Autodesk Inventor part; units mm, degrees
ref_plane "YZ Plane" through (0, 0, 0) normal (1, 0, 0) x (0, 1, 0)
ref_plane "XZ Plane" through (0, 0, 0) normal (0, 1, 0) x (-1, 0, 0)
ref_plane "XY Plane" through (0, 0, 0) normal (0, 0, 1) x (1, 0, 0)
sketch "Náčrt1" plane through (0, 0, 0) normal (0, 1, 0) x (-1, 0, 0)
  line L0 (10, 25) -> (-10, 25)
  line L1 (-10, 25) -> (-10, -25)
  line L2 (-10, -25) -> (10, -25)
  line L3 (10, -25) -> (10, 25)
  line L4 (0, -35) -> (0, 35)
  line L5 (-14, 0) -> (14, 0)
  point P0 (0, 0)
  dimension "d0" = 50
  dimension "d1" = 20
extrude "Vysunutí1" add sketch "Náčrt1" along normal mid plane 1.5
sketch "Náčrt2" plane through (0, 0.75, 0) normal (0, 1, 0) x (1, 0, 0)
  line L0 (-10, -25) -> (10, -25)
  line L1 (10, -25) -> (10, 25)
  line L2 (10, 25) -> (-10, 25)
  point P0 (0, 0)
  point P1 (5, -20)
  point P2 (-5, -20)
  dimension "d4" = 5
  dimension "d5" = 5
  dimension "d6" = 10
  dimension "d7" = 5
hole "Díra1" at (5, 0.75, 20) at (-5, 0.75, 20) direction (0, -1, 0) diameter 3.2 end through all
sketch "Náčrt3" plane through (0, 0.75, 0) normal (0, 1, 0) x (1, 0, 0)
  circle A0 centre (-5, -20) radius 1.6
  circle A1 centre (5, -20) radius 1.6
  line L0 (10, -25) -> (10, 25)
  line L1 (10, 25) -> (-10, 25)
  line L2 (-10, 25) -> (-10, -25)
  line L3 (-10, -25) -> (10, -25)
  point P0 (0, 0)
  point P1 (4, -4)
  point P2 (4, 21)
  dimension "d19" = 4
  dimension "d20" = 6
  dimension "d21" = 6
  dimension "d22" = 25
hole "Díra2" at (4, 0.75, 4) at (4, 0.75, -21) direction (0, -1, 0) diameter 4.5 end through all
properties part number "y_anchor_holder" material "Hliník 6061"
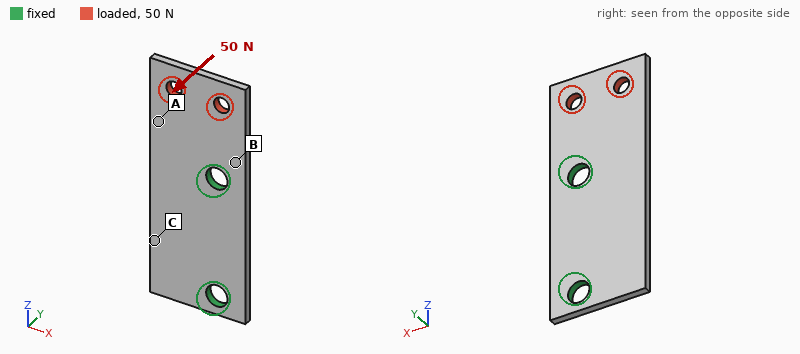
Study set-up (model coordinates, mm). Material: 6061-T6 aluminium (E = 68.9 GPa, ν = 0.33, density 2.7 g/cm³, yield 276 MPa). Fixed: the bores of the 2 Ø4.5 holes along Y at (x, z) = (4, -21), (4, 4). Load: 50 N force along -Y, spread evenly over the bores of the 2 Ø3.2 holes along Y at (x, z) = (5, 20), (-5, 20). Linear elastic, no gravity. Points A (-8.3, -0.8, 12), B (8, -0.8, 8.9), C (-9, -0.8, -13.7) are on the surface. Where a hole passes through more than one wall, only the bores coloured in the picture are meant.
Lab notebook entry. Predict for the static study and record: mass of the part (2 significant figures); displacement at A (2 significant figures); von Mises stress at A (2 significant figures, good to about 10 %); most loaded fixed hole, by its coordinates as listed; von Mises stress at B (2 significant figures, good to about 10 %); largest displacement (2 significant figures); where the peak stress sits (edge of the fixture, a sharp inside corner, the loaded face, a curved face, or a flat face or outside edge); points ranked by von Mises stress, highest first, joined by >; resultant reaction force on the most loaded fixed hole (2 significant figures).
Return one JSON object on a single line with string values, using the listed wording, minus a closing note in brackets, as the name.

{"mass of the part": "3.9 g", "displacement at A": "0.071 mm", "von Mises stress at A": "42 MPa", "most loaded fixed hole, by its coordinates as listed": "(4, 4)", "von Mises stress at B": "81 MPa", "largest displacement": "0.26 mm", "where the peak stress sits": "a flat face or outside edge", "points ranked by von Mises stress, highest first, joined by >": "B > A > C", "resultant reaction force on the most loaded fixed hole": "54 N"}
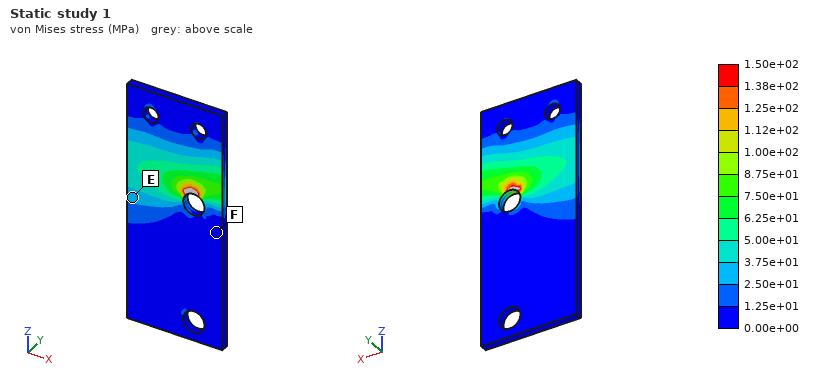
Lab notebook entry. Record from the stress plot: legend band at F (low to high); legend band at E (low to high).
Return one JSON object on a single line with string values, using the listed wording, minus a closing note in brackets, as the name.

{"legend band at F": "0.00e+00 to 1.25e+01 MPa", "legend band at E": "2.50e+01 to 3.75e+01 MPa"}
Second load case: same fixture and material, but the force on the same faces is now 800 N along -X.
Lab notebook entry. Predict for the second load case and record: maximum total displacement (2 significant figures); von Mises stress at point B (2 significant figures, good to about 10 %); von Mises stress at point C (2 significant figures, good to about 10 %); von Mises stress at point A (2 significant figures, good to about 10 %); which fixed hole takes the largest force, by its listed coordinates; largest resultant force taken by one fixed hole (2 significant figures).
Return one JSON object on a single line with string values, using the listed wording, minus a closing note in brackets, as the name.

{"maximum total displacement": "82 µm", "von Mises stress at point B": "82 MPa", "von Mises stress at point C": "21 MPa", "von Mises stress at point A": "58 MPa", "which fixed hole takes the largest force, by its listed coordinates": "(4, 4)", "largest resultant force taken by one fixed hole": "1.2 kN"}
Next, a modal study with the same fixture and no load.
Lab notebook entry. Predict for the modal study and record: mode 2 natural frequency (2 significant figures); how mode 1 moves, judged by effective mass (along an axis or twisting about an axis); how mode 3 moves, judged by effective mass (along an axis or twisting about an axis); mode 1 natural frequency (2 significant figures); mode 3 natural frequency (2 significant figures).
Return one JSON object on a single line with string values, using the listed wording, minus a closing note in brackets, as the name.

{"mode 2 natural frequency": "5600 Hz", "how mode 1 moves, judged by effective mass": "along Y", "how mode 3 moves, judged by effective mass": "along Y", "mode 1 natural frequency": "3000 Hz", "mode 3 natural frequency": "7100 Hz"}
